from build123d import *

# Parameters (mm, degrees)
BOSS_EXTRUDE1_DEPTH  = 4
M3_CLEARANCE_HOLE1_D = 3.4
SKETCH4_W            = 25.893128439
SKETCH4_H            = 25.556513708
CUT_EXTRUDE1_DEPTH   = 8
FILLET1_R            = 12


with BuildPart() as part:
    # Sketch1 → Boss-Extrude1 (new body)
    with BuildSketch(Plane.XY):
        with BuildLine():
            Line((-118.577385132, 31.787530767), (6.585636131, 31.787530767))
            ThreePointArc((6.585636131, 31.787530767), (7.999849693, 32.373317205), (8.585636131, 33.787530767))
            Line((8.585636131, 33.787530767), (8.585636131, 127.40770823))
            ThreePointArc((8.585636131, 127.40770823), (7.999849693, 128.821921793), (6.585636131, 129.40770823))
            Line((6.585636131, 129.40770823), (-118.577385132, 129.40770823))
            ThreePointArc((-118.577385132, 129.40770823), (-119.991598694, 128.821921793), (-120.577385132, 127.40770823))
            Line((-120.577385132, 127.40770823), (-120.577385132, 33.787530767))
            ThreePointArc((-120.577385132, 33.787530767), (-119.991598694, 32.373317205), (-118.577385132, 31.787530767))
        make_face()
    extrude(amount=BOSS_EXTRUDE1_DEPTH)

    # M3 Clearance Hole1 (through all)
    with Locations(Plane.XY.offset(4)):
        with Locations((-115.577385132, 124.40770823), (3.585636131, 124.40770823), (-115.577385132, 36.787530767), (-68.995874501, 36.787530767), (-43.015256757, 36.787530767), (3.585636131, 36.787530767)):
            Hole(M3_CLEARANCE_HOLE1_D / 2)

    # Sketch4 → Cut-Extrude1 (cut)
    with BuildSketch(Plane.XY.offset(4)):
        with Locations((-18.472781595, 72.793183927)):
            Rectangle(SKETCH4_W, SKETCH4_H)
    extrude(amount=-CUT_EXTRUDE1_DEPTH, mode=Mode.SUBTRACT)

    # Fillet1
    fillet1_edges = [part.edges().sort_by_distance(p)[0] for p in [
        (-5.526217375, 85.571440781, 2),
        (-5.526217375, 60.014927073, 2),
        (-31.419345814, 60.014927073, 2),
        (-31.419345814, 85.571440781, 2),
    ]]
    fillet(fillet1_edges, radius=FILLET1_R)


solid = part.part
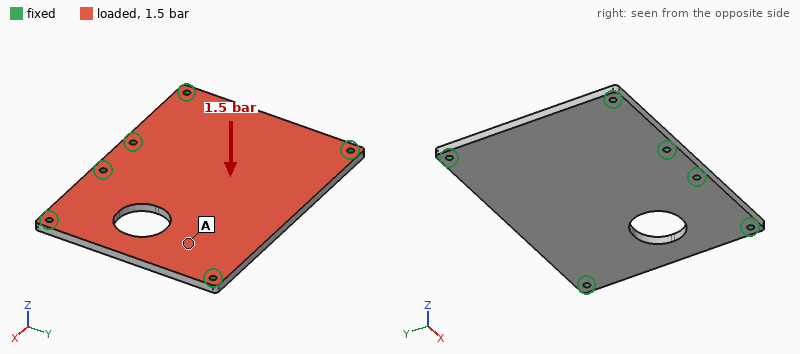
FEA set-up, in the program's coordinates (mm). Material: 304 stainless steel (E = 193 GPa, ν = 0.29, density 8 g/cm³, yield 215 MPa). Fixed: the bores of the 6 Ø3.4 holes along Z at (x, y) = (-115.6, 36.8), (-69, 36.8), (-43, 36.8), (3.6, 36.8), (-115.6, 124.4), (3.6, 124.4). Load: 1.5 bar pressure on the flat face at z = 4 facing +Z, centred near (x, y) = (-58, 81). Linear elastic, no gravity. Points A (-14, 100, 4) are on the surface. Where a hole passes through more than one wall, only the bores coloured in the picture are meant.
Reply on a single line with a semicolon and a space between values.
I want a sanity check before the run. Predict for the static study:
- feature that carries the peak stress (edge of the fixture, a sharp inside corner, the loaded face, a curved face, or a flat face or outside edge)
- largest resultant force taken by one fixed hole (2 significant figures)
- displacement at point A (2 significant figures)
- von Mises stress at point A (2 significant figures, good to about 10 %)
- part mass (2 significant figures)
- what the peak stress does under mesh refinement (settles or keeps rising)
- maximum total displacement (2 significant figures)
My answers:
edge of the fixture; 420 N; 0.048 mm; 20 MPa; 380 g; keeps rising; 0.10 mm
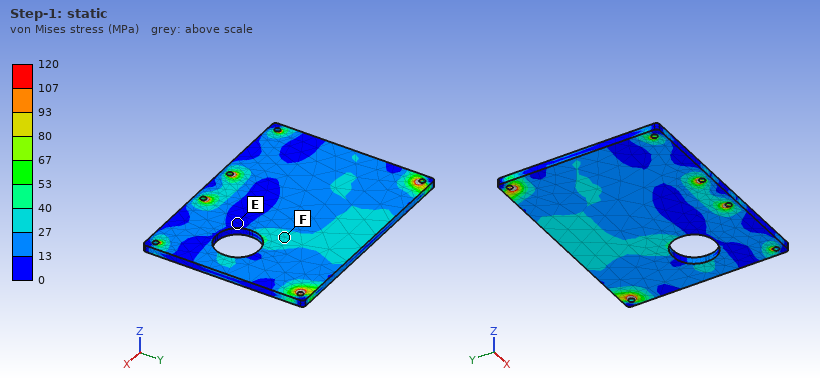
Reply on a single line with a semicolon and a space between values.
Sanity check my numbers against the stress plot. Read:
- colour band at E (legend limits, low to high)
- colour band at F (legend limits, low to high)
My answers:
0 to 13 MPa; 27 to 40 MPa
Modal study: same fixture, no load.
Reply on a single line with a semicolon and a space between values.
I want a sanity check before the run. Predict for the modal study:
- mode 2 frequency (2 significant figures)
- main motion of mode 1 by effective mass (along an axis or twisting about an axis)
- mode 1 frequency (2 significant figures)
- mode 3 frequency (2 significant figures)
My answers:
2400 Hz; along Z; 1300 Hz; 2500 Hz
